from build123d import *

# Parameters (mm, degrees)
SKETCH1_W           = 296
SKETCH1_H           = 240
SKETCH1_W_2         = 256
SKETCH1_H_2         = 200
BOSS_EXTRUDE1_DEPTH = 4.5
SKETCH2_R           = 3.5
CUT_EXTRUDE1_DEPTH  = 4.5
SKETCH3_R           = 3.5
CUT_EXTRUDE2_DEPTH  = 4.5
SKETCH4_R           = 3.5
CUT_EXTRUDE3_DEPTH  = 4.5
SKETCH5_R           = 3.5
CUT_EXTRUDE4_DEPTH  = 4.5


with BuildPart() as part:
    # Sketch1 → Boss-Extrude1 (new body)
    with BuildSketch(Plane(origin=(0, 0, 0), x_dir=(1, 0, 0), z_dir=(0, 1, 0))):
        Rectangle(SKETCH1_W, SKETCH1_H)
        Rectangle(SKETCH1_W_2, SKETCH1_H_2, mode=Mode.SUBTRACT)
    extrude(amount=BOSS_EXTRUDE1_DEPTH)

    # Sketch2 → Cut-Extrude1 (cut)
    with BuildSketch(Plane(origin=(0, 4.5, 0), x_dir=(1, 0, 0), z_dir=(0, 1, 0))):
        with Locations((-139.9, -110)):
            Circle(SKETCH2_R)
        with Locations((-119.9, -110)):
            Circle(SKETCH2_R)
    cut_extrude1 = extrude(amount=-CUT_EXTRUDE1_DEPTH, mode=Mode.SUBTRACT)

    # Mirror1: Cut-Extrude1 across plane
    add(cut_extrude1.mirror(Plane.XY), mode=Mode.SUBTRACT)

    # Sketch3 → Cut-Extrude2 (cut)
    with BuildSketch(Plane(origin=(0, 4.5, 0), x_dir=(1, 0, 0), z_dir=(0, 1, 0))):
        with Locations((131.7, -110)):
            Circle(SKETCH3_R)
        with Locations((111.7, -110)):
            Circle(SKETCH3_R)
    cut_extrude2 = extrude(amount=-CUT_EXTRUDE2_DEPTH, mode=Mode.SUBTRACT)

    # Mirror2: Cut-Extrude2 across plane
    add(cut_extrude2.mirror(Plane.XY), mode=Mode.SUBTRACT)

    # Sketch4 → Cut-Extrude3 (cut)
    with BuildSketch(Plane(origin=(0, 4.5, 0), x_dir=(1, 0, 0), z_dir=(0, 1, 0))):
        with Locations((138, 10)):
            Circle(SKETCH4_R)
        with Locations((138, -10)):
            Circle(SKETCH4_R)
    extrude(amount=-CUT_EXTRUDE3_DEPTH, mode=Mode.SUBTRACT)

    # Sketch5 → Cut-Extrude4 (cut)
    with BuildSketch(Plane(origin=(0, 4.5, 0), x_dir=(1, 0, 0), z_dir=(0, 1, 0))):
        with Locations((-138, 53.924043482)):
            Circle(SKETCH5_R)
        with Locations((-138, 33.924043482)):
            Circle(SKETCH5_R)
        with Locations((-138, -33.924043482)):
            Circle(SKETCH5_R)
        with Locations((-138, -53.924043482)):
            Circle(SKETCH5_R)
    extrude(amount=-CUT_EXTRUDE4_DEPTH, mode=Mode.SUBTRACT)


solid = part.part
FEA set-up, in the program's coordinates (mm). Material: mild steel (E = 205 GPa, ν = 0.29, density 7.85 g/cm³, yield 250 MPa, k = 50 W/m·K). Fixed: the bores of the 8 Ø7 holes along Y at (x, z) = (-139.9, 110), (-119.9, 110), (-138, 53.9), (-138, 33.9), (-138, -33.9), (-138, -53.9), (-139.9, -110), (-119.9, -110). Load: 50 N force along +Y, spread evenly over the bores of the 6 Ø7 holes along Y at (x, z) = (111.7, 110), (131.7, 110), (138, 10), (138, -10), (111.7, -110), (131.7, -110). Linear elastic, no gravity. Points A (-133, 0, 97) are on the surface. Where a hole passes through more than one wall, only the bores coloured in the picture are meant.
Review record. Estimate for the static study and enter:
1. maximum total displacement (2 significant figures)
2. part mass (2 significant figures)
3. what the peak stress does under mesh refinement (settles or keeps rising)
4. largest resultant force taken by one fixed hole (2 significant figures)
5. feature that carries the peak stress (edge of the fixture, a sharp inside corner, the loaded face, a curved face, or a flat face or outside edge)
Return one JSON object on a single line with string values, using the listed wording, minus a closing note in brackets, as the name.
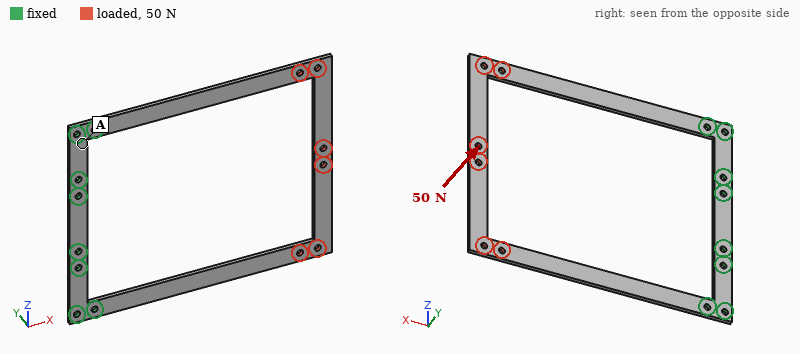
{"maximum total displacement": "4.5 mm", "part mass": "680 g", "what the peak stress does under mesh refinement": "keeps rising", "largest resultant force taken by one fixed hole": "48 N", "feature that carries the peak stress": "edge of the fixture"}
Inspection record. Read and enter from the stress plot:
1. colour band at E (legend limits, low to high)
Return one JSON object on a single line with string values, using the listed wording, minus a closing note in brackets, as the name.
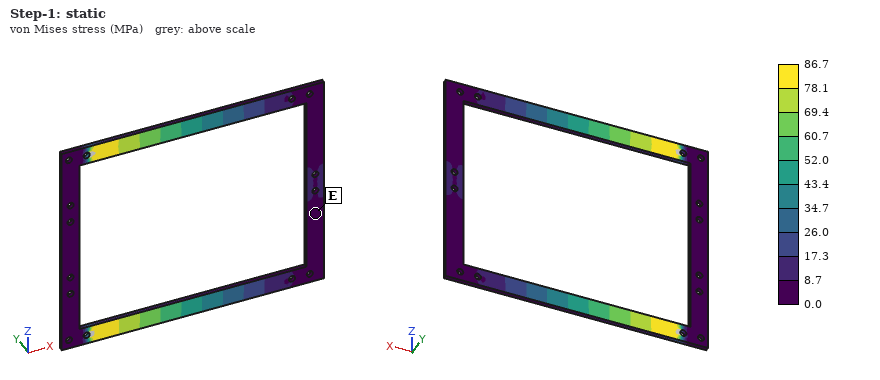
{"colour band at E": "0.0 to 8.7 MPa"}
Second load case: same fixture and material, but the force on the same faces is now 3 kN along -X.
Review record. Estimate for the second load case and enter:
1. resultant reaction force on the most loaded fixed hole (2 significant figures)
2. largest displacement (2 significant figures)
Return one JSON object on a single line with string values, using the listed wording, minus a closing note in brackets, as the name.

{"resultant reaction force on the most loaded fixed hole": "1.4 kN", "largest displacement": "0.21 mm"}
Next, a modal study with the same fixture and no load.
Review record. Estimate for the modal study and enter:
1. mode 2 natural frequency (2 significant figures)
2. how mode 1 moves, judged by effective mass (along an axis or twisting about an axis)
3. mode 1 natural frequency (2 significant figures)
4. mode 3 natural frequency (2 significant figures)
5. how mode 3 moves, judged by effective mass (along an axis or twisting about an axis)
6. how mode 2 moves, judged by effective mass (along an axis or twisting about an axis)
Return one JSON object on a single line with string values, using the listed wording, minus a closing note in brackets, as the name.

{"mode 2 natural frequency": "87 Hz", "how mode 1 moves, judged by effective mass": "along Y", "mode 1 natural frequency": "35 Hz", "mode 3 natural frequency": "240 Hz", "how mode 3 moves, judged by effective mass": "along Z", "how mode 2 moves, judged by effective mass": "twisting about X"}
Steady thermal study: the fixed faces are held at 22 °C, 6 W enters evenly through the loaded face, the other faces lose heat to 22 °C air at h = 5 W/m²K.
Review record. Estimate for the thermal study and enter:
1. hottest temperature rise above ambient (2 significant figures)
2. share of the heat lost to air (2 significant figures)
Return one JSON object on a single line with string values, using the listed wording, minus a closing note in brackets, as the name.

{"hottest temperature rise above ambient": "53 K", "share of the heat lost to air": "82 %"}
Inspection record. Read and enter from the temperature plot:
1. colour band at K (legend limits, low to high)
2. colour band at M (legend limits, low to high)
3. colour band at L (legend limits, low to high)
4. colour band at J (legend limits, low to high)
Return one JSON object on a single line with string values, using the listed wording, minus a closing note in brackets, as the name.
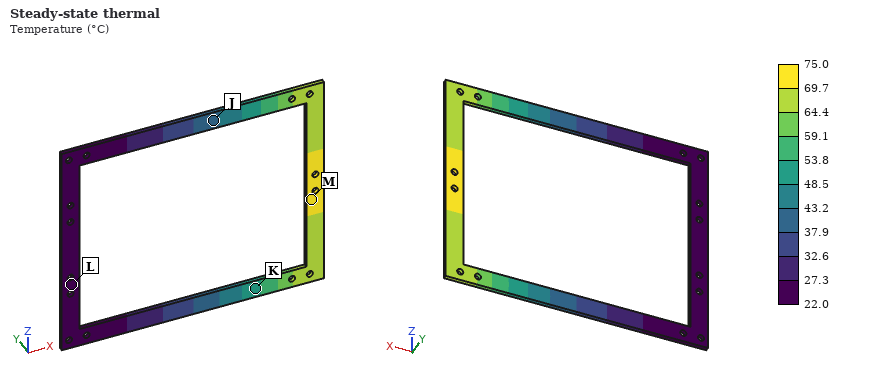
{"colour band at K": "48.5 to 53.8 °C", "colour band at M": "69.7 to 75.0 °C", "colour band at L": "22.0 to 27.3 °C", "colour band at J": "37.9 to 43.2 °C"}
